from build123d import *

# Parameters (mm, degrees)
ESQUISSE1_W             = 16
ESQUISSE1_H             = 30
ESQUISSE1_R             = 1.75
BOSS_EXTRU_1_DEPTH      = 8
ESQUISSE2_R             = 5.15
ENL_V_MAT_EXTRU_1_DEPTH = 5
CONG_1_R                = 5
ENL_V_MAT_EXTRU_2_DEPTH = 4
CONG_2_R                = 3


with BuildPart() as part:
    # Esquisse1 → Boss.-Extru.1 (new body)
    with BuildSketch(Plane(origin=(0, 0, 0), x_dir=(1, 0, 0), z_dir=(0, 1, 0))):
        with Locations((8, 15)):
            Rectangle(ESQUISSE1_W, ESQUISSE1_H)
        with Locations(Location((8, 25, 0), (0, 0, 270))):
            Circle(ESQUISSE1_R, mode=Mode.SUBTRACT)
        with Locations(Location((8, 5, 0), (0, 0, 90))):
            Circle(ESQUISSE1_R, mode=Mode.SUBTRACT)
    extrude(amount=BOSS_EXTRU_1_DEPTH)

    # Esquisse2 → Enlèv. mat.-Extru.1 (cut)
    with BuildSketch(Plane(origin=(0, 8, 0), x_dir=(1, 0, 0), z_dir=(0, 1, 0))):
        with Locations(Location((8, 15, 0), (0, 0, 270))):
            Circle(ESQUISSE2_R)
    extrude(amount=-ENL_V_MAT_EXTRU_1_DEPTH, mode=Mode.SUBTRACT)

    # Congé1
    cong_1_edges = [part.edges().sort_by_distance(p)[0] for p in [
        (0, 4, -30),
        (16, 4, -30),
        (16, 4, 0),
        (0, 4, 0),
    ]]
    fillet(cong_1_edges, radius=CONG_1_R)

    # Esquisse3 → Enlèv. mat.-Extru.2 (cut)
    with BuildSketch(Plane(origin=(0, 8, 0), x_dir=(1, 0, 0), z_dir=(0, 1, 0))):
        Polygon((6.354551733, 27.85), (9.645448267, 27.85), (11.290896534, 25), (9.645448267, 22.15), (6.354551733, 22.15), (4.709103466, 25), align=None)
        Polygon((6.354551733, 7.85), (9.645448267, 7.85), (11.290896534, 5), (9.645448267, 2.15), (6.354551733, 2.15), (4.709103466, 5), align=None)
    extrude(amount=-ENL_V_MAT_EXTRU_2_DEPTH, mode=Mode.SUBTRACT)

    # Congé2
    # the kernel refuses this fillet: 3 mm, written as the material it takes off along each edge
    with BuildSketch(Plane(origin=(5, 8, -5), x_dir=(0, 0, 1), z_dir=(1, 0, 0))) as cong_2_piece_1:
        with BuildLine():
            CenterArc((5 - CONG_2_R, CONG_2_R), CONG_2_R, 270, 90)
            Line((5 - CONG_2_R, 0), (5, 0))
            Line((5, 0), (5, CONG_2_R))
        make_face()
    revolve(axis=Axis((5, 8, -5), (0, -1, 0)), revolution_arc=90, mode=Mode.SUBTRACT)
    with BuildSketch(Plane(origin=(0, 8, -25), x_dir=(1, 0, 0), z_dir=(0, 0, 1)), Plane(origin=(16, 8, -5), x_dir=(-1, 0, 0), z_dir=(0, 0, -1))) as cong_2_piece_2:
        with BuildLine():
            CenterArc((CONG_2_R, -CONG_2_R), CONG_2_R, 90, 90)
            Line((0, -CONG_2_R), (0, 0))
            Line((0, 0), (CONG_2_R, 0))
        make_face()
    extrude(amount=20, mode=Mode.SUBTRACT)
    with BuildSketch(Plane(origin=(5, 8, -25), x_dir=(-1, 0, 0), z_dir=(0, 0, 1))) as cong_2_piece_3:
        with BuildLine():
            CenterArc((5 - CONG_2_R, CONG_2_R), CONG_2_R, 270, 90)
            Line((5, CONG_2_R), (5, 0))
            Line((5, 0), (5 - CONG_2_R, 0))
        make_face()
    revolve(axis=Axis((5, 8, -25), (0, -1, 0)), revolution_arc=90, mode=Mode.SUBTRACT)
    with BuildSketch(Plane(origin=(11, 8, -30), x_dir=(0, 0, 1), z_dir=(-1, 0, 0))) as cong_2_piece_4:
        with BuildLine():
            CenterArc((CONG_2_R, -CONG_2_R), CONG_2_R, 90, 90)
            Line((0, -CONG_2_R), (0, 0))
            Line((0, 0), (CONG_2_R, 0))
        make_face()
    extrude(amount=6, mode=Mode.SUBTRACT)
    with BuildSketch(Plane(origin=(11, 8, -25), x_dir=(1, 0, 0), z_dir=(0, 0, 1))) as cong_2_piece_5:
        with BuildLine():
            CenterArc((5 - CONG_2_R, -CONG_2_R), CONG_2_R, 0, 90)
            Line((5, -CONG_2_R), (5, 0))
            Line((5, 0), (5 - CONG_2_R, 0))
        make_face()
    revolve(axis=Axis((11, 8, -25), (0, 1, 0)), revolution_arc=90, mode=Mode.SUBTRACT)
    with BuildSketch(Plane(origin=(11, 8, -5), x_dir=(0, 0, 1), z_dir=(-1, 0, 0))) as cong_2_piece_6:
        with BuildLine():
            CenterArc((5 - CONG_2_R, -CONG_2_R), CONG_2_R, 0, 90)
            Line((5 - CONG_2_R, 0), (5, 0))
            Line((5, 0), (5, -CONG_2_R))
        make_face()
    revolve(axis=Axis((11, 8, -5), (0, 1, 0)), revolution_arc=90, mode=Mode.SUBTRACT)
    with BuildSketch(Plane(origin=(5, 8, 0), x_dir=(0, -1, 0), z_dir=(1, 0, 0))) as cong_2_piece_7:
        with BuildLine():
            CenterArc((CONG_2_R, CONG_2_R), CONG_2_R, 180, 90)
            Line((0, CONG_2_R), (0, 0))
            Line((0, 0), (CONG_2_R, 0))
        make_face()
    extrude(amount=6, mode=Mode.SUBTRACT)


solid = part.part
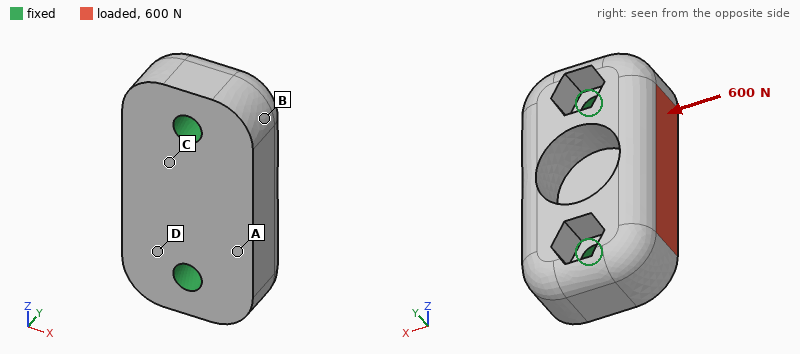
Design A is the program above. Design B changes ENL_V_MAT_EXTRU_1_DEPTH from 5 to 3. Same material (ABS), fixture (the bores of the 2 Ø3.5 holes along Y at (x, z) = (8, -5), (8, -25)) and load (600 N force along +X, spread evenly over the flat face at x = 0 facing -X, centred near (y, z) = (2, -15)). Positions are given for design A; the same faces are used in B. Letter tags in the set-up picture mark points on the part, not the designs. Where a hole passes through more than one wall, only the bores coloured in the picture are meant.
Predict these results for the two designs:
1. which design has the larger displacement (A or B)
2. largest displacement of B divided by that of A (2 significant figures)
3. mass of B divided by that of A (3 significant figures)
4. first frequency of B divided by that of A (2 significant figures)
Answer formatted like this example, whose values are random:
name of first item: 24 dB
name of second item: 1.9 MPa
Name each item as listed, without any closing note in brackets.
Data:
which design has the larger displacement: A
largest displacement of B divided by that of A: 0.83
mass of B divided by that of A: 1.06
first frequency of B divided by that of A: 0.99
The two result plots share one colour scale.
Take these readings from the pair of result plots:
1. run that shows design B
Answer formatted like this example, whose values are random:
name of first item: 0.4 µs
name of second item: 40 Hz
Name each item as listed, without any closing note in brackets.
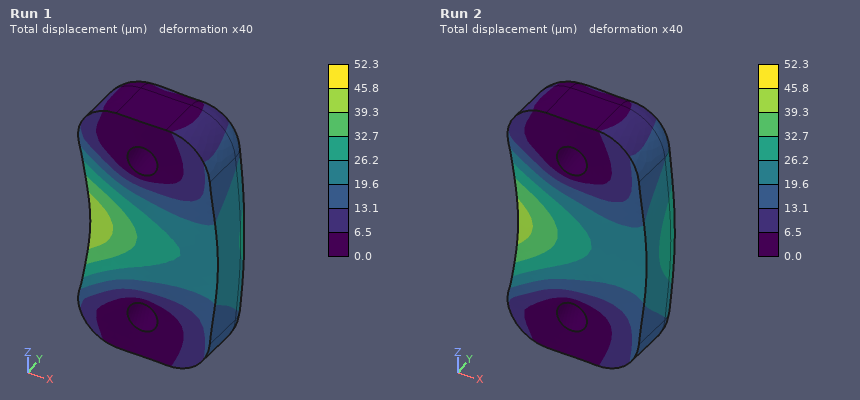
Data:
run that shows design B: Run 2
